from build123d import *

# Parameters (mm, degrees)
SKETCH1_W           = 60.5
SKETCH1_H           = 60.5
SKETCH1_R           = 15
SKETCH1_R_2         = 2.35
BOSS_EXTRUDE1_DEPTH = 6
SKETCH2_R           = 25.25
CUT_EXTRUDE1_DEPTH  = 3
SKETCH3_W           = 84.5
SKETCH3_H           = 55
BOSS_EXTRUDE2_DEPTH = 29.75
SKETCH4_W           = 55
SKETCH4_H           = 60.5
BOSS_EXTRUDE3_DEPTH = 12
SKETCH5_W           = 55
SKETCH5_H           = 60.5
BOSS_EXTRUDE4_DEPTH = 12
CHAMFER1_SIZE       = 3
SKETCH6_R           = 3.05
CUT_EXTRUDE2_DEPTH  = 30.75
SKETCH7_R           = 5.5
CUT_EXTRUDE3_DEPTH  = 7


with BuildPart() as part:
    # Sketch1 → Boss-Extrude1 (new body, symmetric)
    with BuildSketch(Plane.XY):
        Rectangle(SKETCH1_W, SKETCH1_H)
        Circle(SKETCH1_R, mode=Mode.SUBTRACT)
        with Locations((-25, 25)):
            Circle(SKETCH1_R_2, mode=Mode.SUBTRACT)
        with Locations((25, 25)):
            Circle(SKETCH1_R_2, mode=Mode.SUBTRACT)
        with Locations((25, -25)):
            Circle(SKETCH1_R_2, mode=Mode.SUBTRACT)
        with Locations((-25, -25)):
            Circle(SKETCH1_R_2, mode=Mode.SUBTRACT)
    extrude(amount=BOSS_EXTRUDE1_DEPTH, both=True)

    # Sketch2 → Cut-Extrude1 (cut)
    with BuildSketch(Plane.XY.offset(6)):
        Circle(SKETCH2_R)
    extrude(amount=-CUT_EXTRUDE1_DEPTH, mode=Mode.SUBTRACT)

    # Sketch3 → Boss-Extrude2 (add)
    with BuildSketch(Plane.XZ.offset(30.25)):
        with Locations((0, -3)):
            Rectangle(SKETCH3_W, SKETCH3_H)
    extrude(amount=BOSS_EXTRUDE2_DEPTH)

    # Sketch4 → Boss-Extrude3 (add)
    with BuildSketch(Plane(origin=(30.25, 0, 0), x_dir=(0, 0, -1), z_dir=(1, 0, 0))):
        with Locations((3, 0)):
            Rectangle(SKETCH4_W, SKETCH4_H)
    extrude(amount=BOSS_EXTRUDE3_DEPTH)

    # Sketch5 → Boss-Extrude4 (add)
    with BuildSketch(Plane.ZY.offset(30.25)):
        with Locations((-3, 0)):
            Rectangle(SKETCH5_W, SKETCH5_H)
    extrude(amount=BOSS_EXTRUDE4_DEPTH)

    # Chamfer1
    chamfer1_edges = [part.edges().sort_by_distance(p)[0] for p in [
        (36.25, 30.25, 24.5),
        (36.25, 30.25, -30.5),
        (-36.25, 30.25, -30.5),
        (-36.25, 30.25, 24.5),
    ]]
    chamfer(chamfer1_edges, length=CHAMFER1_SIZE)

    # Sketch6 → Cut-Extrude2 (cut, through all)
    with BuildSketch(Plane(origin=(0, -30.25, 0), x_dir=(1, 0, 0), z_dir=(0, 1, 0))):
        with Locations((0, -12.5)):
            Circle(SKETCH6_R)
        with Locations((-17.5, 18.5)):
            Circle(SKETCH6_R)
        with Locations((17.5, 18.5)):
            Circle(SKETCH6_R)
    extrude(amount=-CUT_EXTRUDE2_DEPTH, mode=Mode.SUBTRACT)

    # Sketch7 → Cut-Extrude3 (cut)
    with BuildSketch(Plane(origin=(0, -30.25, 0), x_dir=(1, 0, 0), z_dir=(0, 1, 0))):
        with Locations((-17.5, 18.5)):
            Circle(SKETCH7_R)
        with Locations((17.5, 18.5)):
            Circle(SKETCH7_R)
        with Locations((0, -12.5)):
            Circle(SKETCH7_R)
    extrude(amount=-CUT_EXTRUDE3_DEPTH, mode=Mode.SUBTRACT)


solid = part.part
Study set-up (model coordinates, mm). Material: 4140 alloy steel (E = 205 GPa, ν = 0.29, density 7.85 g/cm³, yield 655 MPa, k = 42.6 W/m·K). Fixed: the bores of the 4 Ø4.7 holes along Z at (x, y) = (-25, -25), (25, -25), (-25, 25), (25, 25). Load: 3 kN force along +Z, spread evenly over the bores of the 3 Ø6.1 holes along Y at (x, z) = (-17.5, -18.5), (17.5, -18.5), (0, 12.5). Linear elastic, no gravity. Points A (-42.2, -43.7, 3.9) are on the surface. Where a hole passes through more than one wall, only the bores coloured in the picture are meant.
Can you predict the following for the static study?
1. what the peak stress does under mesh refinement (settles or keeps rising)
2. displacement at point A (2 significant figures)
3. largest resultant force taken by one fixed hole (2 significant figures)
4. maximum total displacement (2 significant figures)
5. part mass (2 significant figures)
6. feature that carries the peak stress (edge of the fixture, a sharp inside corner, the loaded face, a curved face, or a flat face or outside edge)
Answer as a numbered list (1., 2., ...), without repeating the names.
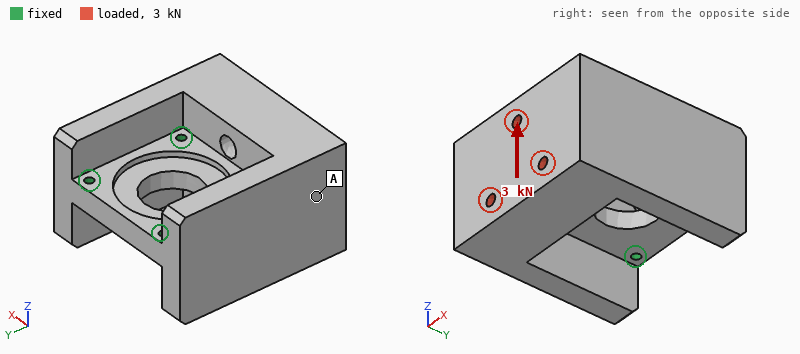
1. keeps rising
2. 1.8 µm
3. 2.1 kN
4. 3.8 µm
5. 1.9 kg
6. edge of the fixture
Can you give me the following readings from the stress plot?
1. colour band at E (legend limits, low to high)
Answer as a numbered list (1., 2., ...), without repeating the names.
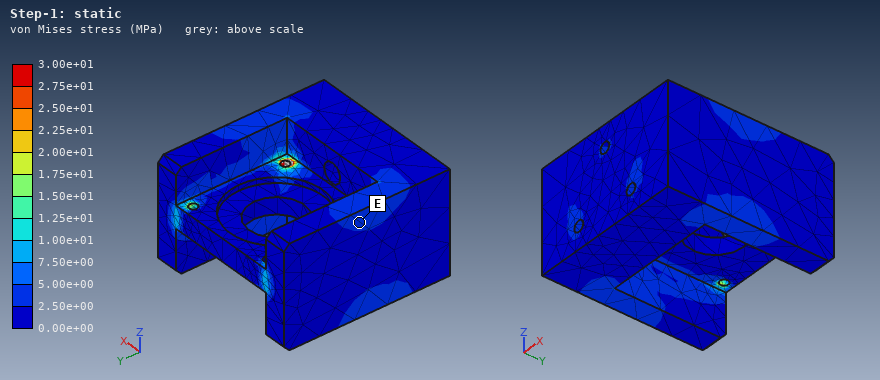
1. 2.50e+00 to 5.00e+00 MPa
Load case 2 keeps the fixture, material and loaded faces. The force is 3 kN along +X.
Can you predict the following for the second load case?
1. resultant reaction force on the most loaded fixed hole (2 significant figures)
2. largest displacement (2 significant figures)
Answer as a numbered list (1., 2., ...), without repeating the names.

1. 1.9 kN
2. 1.5 µm
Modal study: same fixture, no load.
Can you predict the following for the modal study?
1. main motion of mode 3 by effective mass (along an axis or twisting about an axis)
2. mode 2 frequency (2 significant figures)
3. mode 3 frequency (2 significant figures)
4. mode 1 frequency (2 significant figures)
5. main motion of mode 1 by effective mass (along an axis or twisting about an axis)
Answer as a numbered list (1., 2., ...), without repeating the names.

1. along Z
2. 6200 Hz
3. 7600 Hz
4. 5100 Hz
5. along Z
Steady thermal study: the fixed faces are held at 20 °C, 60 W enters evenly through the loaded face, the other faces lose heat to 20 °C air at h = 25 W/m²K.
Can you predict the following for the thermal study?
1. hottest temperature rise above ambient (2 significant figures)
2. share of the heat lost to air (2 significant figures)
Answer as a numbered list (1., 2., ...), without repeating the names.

1. 27 K
2. 18 %
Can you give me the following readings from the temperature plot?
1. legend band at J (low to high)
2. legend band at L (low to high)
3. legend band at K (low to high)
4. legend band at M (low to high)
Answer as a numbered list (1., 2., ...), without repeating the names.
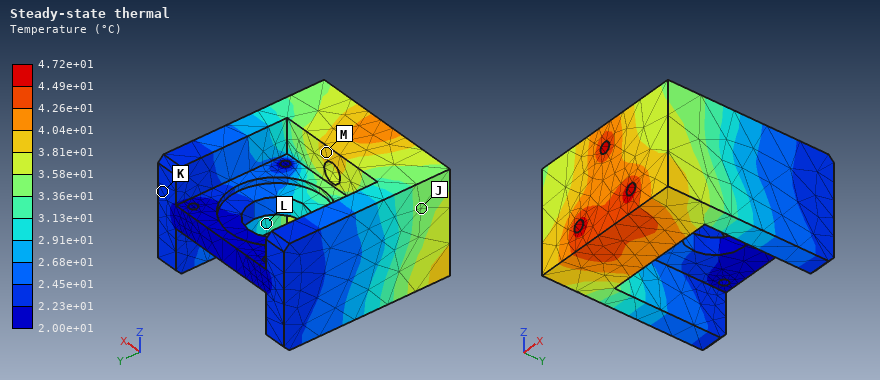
1. 3.36e+01 to 3.58e+01 °C
2. 2.91e+01 to 3.13e+01 °C
3. 2.23e+01 to 2.45e+01 °C
4. 3.81e+01 to 4.04e+01 °C
